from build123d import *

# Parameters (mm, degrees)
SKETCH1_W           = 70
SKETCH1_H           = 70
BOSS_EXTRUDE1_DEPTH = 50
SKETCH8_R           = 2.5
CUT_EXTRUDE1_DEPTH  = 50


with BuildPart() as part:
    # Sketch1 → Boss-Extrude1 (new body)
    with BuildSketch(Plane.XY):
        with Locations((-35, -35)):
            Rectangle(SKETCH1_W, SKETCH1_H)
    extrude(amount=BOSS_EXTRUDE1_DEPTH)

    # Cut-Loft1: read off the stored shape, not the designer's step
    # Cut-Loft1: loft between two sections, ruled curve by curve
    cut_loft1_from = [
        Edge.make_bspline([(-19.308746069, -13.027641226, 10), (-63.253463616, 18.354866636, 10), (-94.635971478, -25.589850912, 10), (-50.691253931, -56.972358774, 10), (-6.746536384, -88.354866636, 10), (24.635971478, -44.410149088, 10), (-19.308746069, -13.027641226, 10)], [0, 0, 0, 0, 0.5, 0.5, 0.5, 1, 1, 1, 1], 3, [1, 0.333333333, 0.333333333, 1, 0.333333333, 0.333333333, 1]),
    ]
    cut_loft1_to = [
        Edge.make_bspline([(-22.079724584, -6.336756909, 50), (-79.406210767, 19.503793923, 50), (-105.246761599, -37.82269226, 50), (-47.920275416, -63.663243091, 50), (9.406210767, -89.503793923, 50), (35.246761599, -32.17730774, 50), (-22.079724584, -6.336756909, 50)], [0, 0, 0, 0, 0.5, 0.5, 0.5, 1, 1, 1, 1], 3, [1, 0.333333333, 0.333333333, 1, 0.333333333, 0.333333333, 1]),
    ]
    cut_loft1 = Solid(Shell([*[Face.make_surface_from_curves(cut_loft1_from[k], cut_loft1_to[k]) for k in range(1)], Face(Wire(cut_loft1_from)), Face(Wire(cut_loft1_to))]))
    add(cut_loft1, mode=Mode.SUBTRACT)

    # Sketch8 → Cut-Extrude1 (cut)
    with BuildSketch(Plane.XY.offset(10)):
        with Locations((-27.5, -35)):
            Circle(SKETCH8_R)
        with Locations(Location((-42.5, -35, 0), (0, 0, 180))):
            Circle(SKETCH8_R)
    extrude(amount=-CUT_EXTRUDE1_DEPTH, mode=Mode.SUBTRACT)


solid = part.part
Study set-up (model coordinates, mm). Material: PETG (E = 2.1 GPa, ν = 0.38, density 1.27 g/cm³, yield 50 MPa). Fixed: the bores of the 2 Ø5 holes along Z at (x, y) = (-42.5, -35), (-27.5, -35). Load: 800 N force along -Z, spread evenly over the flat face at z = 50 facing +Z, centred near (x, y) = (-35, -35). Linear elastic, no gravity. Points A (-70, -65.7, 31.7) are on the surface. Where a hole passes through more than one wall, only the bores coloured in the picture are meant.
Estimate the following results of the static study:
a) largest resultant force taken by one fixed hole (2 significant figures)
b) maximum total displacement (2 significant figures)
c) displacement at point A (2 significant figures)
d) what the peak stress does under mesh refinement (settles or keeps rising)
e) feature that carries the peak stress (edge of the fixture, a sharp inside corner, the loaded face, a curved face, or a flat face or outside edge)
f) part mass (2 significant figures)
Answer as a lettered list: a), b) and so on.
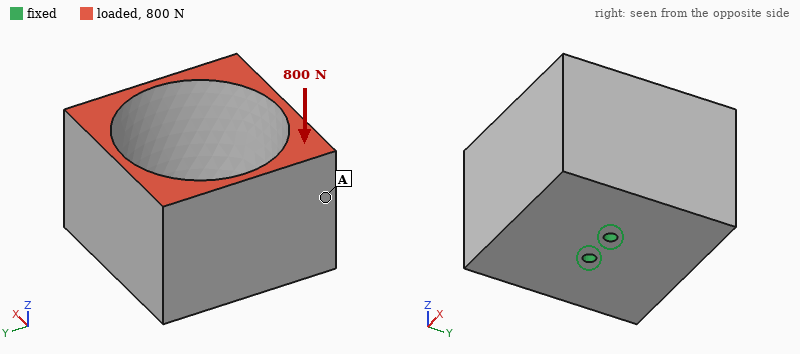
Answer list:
a) 400 N
b) 95 µm
c) 90 µm
d) keeps rising
e) edge of the fixture
f) 170 g
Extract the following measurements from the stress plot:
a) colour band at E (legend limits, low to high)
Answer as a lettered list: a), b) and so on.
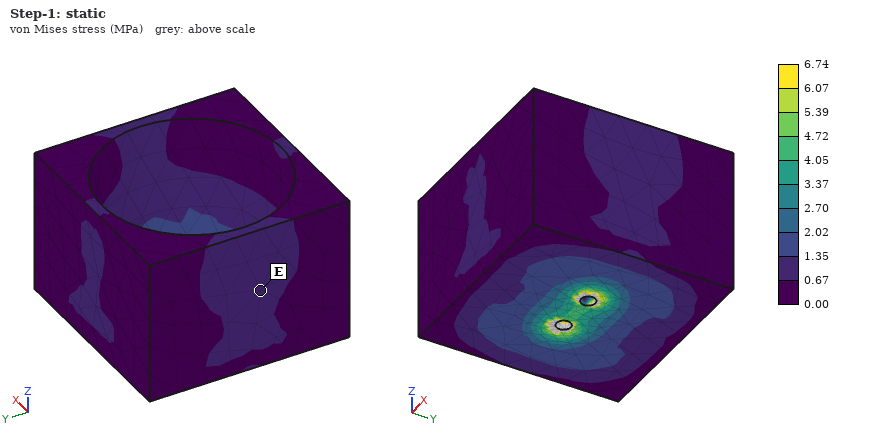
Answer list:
a) 0.67 to 1.35 MPa
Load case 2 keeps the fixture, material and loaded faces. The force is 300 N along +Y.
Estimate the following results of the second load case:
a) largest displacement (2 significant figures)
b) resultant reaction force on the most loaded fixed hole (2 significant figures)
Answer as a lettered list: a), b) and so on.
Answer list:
a) 0.61 mm
b) 150 N
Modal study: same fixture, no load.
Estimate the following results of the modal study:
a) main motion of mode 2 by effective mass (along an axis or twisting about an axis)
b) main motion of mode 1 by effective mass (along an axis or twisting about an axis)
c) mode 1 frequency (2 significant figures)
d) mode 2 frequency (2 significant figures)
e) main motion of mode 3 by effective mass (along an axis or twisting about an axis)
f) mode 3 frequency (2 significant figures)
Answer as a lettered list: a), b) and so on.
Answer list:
a) along X
b) along Y
c) 440 Hz
d) 580 Hz
e) twisting about Z
f) 800 Hz
